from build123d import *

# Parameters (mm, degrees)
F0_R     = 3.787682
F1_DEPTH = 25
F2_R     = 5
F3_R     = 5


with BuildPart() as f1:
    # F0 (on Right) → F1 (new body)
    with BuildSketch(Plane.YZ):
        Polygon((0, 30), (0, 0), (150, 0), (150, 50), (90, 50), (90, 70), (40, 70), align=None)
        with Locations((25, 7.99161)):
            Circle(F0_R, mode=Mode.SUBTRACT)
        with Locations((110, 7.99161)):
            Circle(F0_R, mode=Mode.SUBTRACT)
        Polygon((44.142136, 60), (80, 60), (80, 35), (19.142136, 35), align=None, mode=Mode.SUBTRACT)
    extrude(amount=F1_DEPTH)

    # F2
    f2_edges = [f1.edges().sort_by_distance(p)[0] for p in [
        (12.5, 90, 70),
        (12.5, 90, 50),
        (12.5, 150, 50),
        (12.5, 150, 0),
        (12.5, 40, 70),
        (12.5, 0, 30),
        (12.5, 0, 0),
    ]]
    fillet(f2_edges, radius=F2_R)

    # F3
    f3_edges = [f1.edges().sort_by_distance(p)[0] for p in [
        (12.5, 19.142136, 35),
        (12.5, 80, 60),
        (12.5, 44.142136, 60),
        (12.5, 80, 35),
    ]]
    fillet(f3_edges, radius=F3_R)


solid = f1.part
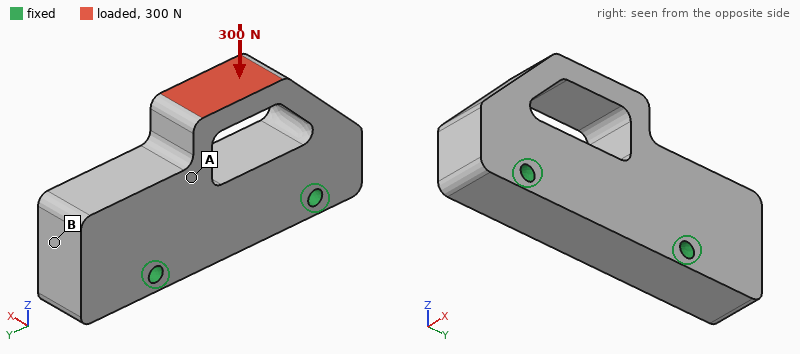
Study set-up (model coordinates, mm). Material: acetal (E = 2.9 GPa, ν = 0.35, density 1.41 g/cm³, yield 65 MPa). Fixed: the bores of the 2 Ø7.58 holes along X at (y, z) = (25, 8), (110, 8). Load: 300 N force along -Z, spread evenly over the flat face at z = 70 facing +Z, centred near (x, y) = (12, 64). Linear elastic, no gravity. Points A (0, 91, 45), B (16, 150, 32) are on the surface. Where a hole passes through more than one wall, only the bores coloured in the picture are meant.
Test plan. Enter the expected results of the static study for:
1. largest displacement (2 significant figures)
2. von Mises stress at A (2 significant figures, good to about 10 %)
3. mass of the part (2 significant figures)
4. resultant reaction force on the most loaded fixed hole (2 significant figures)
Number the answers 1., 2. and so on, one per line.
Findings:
1. 42 µm
2. 0.48 MPa
3. 250 g
4. 160 N
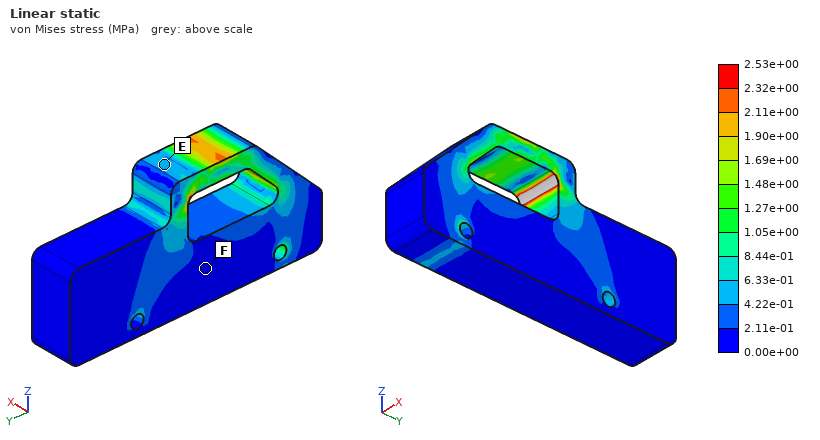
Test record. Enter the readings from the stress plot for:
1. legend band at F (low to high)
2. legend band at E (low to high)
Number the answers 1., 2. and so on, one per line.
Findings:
1. 0.00e+00 to 2.11e-01 MPa
2. 4.22e-01 to 6.33e-01 MPa
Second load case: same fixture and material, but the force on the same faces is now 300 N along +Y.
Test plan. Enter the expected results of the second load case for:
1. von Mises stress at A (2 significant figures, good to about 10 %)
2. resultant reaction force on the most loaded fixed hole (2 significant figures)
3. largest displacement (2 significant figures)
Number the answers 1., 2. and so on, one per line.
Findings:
1. 0.85 MPa
2. 260 N
3. 49 µm
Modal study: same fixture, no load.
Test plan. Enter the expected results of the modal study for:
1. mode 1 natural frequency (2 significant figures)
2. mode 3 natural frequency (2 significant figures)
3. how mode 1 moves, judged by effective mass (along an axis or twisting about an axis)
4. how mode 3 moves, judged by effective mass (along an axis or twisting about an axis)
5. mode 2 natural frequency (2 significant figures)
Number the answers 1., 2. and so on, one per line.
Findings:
1. 1200 Hz
2. 2000 Hz
3. along X
4. along Y
5. 1800 Hz
